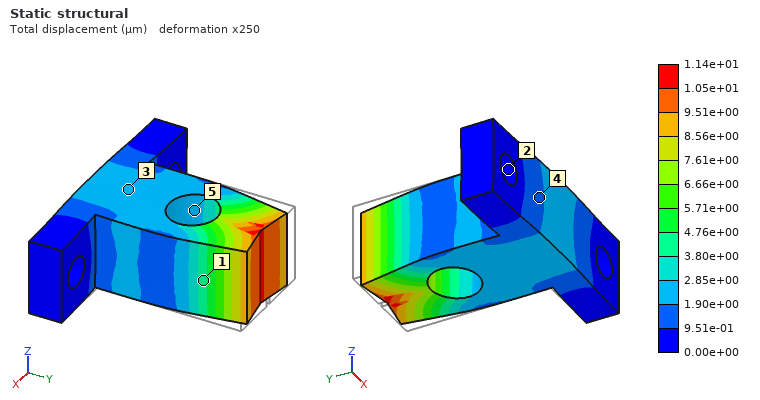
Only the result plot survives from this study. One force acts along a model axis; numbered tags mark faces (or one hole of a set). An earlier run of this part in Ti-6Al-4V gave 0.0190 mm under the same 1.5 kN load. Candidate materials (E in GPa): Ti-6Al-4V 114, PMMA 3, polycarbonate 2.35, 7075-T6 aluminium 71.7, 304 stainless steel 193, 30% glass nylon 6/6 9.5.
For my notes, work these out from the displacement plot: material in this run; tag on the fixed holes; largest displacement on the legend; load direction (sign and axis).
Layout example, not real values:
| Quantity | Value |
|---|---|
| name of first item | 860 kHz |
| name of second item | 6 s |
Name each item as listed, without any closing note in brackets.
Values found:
| Quantity | Value |
|---|---|
| material in this run | 304 stainless steel |
| tag on the fixed holes | 2 |
| largest displacement on the legend | 1.14e+01 µm |
| load direction | -Y |
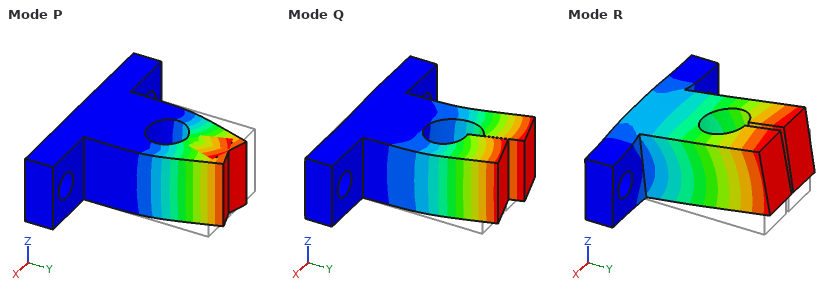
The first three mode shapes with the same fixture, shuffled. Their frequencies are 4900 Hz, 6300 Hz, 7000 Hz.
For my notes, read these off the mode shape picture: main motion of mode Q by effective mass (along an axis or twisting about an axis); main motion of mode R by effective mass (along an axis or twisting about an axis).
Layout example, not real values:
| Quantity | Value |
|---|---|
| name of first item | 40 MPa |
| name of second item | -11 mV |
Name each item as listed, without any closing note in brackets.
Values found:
| Quantity | Value |
|---|---|
| main motion of mode Q by effective mass | along X |
| main motion of mode R by effective mass | along Z |
